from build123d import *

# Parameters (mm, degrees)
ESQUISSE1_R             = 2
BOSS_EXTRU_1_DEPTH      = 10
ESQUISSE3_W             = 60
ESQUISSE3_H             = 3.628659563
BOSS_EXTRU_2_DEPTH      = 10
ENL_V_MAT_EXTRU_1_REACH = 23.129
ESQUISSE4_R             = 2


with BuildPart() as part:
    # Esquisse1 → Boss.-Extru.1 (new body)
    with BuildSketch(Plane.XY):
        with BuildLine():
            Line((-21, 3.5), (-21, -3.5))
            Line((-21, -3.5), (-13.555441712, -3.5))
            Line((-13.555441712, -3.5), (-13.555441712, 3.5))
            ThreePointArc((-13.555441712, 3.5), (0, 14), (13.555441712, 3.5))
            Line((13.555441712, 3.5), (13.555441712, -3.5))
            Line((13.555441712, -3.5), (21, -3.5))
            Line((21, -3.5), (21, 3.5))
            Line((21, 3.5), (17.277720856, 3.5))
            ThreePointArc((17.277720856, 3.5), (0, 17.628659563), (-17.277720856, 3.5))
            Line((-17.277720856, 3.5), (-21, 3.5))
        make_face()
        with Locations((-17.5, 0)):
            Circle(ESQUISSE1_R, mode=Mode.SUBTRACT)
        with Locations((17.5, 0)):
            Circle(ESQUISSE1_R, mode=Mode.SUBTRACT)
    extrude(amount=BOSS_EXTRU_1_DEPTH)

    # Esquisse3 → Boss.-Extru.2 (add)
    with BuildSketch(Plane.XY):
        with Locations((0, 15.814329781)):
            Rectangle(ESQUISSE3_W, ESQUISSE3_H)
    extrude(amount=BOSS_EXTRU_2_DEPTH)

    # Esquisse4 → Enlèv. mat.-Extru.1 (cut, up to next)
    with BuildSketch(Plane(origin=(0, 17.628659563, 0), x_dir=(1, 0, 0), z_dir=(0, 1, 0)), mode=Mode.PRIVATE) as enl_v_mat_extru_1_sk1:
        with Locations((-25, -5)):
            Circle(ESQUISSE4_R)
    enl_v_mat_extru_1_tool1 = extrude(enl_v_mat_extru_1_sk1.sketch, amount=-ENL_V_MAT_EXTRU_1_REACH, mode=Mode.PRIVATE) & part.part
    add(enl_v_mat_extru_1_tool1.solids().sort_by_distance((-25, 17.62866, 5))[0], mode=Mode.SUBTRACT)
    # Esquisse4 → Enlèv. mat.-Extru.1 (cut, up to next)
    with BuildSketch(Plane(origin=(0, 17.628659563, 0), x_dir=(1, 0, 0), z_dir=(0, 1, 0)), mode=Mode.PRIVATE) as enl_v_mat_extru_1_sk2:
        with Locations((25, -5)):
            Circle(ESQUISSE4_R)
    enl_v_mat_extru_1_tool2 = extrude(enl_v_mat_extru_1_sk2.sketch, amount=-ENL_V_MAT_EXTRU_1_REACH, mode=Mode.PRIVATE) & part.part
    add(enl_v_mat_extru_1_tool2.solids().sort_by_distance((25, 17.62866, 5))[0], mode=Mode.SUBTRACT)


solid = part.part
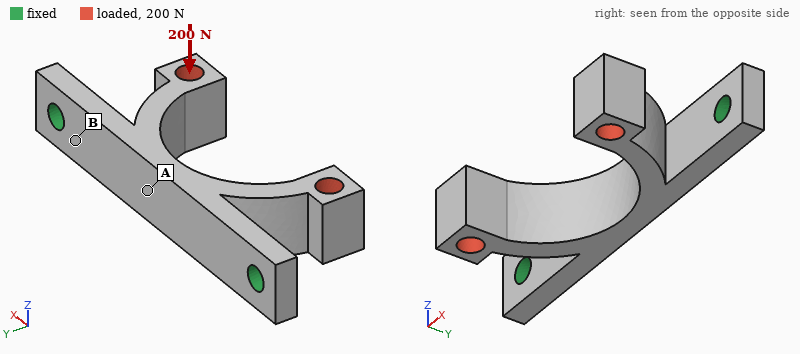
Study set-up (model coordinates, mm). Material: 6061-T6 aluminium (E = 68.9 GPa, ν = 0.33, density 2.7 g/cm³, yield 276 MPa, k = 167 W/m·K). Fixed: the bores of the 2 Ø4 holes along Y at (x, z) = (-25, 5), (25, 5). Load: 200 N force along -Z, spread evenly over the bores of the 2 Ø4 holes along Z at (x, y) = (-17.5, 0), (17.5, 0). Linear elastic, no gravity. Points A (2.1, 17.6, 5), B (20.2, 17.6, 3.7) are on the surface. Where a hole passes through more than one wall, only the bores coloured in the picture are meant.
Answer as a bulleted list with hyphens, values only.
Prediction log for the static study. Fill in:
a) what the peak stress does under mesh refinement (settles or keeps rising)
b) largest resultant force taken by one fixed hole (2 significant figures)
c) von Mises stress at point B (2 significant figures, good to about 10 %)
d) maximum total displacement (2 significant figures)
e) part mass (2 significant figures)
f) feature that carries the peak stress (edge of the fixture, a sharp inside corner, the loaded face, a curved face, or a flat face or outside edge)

- keeps rising
- 100 N
- 58 MPa
- 0.14 mm
- 11 g
- edge of the fixture
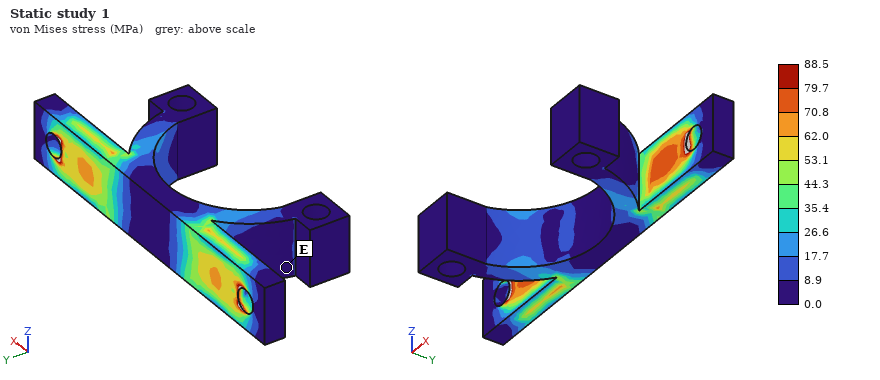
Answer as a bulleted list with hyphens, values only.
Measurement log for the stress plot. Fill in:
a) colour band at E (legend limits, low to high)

- 0.0 to 8.9 MPa
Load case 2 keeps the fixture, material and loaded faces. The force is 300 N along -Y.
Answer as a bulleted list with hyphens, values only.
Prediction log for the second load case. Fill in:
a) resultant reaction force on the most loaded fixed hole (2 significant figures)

- 150 N
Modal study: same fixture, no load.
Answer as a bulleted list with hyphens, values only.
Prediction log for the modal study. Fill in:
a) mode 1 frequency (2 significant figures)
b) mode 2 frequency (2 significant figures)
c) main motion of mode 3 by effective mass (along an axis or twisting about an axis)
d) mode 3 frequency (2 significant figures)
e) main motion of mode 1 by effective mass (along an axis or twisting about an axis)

- 3900 Hz
- 4600 Hz
- along X
- 5000 Hz
- along Z
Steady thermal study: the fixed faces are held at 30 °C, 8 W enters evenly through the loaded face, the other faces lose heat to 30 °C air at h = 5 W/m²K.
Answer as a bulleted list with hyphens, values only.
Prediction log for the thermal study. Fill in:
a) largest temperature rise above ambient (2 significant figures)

- 21 K
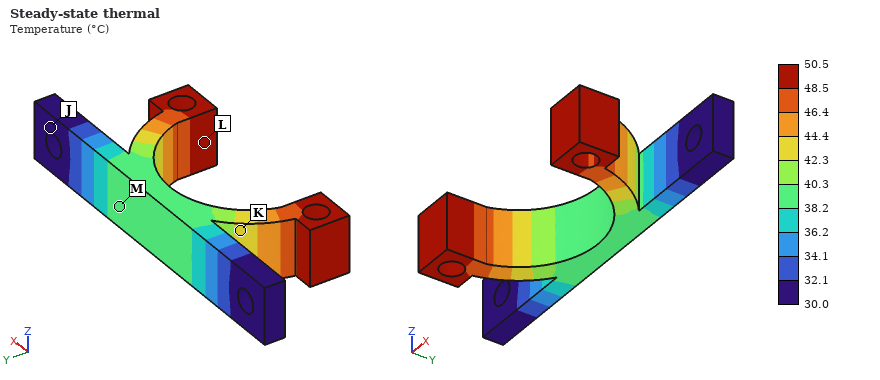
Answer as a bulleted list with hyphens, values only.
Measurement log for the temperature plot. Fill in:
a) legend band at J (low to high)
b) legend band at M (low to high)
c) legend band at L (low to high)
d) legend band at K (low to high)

- 30.0 to 32.1 °C
- 38.2 to 40.3 °C
- 48.5 to 50.5 °C
- 42.3 to 44.4 °C
